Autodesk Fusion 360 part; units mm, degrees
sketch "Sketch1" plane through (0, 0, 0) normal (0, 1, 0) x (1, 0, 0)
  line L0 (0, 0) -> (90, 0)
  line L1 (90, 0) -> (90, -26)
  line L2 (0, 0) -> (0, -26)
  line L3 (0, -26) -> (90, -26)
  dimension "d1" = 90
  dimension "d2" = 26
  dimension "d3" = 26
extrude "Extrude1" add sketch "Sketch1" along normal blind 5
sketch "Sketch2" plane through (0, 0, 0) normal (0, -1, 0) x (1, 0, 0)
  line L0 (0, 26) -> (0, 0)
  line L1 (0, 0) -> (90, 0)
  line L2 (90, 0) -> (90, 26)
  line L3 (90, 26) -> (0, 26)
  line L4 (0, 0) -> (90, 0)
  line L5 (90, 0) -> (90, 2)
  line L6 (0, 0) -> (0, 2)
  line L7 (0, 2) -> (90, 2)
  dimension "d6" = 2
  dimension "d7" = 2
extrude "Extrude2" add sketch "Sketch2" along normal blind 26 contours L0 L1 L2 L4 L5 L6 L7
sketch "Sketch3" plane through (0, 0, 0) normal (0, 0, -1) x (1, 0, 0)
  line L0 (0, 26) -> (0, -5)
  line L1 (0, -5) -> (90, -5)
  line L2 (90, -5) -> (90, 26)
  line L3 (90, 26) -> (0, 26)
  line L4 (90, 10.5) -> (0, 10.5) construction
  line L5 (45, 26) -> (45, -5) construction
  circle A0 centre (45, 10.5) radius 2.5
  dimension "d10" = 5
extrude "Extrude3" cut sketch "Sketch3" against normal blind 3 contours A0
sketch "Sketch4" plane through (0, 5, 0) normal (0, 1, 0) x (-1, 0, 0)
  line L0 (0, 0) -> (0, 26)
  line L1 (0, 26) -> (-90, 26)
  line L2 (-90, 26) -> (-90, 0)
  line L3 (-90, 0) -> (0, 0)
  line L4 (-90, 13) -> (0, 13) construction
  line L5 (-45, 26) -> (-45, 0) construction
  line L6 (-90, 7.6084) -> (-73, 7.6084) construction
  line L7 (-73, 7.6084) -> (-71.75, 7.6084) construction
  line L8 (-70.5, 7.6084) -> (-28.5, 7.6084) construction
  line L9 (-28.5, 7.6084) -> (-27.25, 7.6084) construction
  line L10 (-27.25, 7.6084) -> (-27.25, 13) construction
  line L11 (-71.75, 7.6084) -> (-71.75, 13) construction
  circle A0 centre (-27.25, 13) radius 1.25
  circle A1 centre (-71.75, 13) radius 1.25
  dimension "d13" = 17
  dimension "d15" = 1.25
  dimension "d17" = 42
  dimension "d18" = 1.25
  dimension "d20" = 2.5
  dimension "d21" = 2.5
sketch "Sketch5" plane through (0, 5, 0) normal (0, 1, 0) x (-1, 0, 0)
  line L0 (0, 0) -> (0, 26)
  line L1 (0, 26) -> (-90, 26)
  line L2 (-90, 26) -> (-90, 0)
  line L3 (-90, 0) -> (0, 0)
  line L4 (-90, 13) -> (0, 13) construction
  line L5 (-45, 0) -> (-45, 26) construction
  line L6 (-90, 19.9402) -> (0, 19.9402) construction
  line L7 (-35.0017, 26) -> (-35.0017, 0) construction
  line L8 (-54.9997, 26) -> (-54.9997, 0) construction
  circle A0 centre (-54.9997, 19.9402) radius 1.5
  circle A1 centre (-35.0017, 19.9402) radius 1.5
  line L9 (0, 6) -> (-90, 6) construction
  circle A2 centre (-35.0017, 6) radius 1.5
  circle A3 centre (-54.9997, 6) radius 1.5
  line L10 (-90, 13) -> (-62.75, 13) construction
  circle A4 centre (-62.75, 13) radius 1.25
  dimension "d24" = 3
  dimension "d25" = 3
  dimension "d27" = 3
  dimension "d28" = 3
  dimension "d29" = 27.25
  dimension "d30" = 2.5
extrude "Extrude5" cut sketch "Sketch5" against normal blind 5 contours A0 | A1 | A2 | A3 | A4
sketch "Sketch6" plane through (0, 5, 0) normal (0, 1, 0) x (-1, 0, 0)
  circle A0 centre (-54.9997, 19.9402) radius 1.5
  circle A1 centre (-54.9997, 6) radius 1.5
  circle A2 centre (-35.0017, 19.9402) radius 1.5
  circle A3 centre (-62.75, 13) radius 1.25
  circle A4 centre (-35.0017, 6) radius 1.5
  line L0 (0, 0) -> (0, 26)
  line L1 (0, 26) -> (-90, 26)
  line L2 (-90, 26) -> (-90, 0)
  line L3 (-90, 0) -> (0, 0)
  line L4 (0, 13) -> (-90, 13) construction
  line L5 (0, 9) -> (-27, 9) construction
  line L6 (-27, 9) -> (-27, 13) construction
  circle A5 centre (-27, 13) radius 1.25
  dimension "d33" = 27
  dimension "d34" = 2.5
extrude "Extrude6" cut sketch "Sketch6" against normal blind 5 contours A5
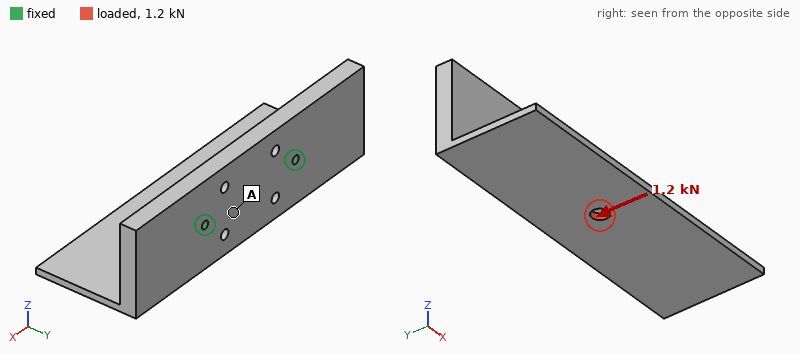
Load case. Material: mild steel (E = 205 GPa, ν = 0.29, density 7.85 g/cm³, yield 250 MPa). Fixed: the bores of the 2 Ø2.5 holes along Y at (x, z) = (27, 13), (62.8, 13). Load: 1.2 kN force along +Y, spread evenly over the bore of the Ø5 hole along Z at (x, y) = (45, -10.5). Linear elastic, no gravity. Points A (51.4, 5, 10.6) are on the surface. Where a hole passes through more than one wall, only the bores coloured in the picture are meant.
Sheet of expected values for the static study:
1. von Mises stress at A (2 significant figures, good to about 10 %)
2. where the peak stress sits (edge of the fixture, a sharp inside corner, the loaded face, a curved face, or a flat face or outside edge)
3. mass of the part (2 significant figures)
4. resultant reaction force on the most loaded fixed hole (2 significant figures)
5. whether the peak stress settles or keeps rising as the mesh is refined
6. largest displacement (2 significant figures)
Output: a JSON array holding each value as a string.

["23 MPa", "edge of the fixture", "130 g", "620 N", "keeps rising", "37 µm"]
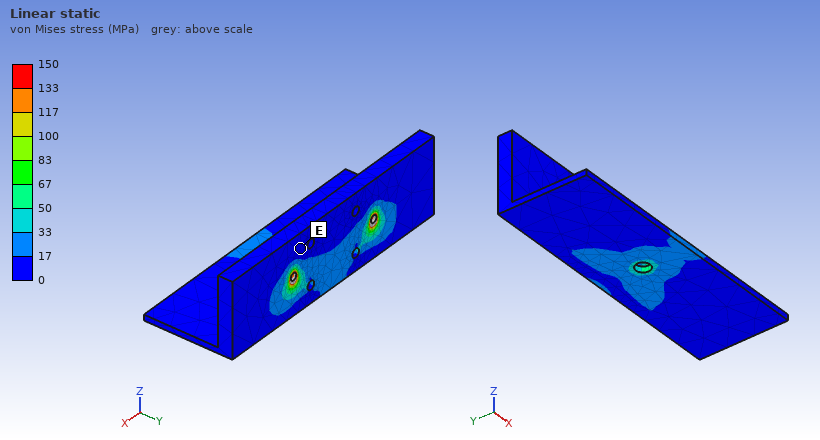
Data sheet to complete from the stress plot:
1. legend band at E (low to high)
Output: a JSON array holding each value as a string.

["0 to 17 MPa"]
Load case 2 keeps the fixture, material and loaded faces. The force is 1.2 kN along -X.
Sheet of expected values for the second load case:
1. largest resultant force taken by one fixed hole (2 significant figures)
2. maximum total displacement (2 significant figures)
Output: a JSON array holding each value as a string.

["800 N", "23 µm"]
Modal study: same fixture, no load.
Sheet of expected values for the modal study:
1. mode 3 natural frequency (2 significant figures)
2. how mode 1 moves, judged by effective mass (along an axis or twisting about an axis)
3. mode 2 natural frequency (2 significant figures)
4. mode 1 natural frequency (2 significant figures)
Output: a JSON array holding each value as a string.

["4000 Hz", "along Z", "2600 Hz", "2100 Hz"]
